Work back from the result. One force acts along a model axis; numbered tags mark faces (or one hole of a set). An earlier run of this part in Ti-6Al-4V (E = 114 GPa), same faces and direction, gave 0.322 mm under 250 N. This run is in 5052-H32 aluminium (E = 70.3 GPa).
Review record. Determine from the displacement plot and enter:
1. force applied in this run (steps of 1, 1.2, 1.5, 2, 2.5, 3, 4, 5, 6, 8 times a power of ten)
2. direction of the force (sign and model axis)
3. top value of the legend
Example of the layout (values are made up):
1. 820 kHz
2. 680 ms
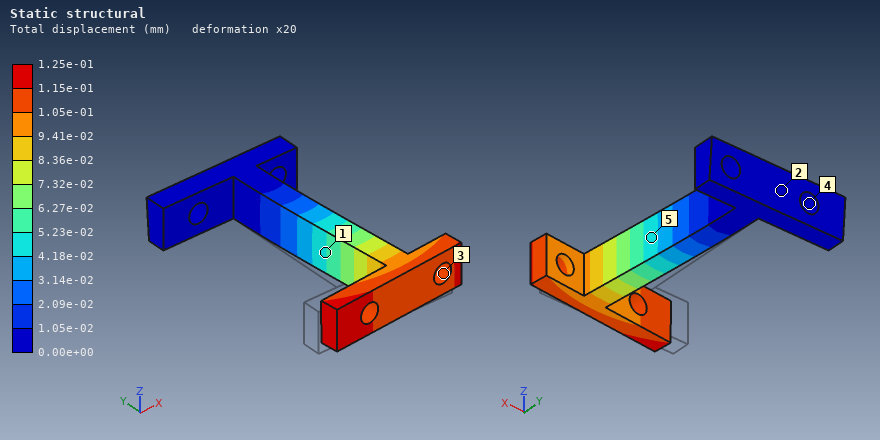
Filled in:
1. 60 N
2. +X
3. 1.25e-01 mm
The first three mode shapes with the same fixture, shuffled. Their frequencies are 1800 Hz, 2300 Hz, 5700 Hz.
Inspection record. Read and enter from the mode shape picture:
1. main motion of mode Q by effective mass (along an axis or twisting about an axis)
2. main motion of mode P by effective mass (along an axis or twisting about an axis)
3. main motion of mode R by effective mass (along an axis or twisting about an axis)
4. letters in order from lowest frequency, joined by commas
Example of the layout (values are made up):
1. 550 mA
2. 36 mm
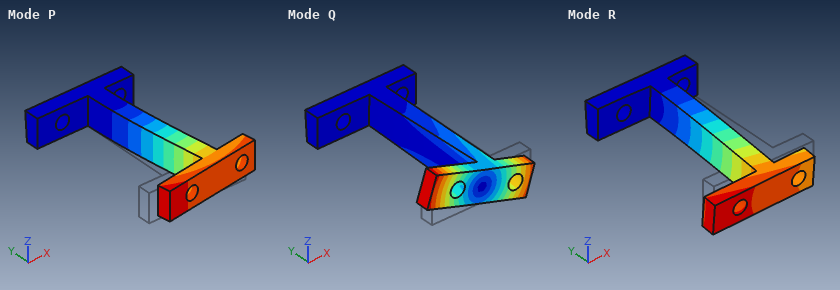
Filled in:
1. twisting about Y
2. along X
3. along Z
4. P, R, Q
